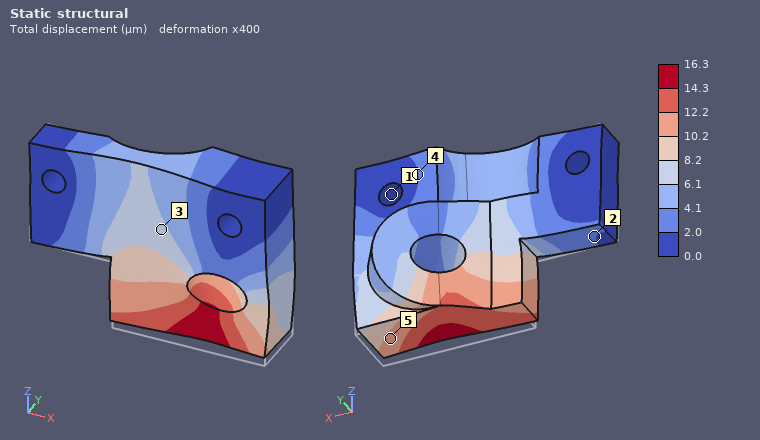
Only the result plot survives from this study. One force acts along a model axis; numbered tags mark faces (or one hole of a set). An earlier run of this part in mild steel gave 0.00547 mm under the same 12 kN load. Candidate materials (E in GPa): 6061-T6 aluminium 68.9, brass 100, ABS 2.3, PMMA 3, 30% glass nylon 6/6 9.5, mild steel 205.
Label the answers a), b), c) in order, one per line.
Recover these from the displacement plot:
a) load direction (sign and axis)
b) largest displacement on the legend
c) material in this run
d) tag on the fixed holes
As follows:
a) +Z
b) 16.3 µm
c) 6061-T6 aluminium
d) 1
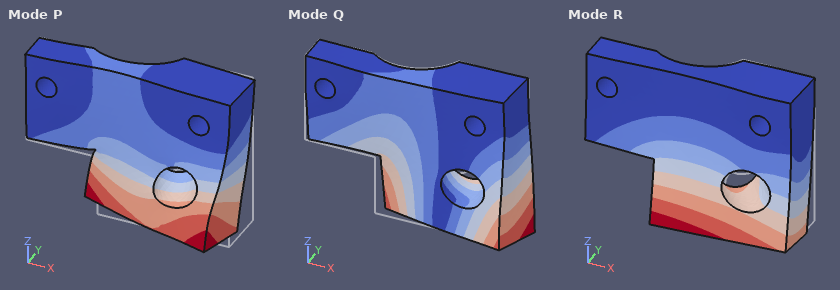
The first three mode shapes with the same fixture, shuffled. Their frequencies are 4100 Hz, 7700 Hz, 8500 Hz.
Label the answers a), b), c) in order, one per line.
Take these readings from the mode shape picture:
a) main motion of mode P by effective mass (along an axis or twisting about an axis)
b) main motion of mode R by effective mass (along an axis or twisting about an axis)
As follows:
a) along X
b) along Y
